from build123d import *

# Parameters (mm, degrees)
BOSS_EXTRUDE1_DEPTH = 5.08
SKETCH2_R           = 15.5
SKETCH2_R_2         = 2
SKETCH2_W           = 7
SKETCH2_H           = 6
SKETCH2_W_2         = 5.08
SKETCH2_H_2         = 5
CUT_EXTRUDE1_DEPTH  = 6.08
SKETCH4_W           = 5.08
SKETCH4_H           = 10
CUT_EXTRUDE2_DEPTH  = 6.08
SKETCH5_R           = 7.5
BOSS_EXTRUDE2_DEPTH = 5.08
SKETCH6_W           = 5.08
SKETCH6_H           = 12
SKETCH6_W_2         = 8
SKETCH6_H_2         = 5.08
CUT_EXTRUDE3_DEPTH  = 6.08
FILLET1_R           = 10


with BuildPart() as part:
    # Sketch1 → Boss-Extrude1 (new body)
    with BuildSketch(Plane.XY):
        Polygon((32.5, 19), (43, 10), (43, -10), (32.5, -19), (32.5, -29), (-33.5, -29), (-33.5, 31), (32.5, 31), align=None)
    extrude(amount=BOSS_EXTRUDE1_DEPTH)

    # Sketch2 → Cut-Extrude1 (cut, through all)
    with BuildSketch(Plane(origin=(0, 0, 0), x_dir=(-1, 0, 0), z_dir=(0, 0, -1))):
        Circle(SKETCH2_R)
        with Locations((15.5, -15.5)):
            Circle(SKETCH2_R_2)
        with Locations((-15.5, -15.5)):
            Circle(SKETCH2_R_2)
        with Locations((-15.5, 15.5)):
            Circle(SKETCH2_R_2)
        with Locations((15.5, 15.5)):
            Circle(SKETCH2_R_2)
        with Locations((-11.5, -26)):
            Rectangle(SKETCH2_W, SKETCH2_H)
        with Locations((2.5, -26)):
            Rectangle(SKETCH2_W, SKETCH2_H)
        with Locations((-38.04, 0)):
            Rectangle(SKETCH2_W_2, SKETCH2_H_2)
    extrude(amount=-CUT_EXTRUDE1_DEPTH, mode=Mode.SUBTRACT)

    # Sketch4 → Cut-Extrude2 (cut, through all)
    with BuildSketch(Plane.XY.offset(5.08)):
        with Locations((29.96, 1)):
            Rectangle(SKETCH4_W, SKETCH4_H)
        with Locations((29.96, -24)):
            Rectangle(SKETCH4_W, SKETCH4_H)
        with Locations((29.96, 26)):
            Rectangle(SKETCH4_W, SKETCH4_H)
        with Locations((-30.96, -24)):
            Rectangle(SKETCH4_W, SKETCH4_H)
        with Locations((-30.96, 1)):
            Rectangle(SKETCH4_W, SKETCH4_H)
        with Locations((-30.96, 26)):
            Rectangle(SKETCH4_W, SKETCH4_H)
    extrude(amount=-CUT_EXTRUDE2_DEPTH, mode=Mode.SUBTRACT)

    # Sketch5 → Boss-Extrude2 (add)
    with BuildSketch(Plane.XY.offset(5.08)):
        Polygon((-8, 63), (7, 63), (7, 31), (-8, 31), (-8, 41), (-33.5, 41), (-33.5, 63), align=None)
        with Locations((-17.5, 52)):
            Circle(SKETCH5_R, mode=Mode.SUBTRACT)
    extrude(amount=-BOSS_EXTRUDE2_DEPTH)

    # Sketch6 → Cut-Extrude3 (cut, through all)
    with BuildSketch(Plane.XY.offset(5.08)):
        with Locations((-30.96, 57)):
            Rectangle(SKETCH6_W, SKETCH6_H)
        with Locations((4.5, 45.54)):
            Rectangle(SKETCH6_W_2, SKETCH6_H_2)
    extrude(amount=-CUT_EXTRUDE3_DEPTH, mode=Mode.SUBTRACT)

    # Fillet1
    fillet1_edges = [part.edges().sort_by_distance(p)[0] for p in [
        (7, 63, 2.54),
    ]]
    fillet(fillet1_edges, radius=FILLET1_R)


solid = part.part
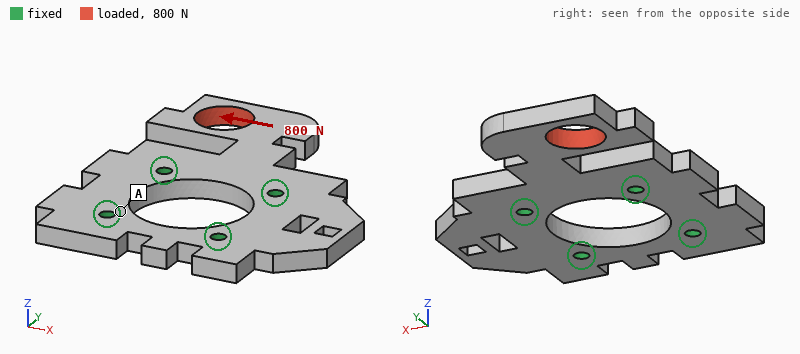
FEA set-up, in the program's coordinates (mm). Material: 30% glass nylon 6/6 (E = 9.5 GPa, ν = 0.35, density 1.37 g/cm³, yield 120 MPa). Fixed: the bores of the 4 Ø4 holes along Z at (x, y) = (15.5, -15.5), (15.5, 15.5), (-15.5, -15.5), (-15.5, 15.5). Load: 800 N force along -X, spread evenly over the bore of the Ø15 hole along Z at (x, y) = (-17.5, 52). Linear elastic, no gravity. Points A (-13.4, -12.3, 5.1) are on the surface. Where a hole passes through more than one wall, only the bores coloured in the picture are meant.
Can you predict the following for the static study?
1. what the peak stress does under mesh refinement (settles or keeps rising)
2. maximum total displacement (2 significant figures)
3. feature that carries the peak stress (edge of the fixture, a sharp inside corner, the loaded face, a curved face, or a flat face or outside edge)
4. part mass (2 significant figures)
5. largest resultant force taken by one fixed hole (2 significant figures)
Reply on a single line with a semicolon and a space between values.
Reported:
keeps rising; 1.4 mm; a sharp inside corner; 26 g; 950 N
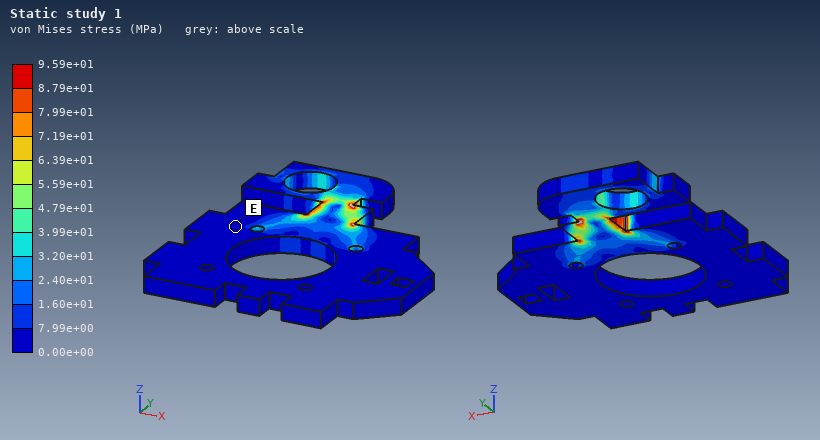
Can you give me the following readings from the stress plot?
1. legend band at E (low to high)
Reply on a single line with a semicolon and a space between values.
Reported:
0.00e+00 to 7.99e+00 MPa
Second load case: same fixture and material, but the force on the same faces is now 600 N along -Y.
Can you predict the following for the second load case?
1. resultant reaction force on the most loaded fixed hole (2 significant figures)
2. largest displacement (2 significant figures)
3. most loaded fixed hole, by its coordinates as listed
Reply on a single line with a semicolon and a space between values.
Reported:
670 N; 1.3 mm; (-15.5, 15.5)
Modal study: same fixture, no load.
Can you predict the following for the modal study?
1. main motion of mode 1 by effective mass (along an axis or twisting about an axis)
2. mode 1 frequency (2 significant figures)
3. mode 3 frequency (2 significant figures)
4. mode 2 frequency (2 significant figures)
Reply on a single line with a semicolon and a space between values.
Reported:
along Z; 770 Hz; 1900 Hz; 1600 Hz
